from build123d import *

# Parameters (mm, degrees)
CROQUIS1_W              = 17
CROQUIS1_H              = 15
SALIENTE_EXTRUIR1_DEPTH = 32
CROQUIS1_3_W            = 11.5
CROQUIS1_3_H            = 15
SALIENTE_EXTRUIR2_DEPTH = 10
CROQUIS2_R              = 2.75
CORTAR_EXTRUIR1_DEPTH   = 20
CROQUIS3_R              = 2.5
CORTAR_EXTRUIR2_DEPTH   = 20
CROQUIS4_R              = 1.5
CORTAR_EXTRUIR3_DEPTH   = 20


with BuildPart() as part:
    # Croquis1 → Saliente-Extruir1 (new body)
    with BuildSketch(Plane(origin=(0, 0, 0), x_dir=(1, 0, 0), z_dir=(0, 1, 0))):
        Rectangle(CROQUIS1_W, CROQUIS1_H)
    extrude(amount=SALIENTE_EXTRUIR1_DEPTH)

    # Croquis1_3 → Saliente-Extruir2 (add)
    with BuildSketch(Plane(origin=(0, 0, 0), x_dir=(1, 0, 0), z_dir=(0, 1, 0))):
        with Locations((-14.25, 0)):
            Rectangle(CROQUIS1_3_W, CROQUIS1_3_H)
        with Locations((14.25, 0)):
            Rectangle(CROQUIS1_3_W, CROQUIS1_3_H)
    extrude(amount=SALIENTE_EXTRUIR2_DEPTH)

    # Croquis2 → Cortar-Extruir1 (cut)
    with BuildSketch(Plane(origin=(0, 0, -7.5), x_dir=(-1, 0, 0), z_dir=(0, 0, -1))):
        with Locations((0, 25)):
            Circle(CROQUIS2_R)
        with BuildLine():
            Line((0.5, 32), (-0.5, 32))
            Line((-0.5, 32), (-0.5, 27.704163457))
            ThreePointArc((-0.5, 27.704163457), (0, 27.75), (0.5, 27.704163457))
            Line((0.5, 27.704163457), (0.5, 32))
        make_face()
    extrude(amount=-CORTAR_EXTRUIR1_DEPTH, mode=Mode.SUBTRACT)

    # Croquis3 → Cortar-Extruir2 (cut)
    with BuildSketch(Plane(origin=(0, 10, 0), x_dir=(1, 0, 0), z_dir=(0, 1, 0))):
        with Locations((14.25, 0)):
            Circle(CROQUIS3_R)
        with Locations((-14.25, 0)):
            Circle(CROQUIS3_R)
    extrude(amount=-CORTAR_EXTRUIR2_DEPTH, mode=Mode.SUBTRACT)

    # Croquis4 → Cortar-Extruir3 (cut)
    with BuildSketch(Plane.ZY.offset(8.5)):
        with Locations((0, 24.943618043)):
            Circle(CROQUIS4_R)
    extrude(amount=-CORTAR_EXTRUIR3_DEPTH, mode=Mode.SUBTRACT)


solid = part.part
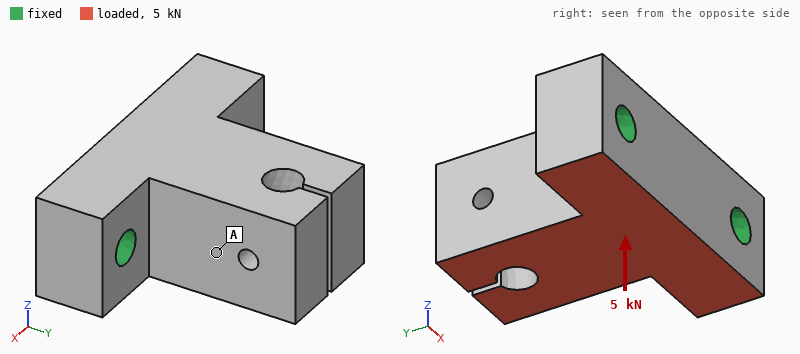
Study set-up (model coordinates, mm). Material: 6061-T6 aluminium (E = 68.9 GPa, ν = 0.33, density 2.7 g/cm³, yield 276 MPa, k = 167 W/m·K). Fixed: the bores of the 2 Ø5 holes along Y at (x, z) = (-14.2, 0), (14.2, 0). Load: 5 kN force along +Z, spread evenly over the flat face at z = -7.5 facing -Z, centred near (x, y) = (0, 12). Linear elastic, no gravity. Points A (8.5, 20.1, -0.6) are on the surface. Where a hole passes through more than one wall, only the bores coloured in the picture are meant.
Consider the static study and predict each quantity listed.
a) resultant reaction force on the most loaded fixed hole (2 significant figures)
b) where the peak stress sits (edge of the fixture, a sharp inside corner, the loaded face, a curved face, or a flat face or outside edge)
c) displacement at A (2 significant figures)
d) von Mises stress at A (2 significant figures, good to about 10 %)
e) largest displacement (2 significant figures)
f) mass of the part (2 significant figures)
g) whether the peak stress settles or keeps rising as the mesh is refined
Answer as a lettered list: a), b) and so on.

a) 2.5 kN
b) edge of the fixture
c) 39 µm
d) 17 MPa
e) 75 µm
f) 29 g
g) keeps rising
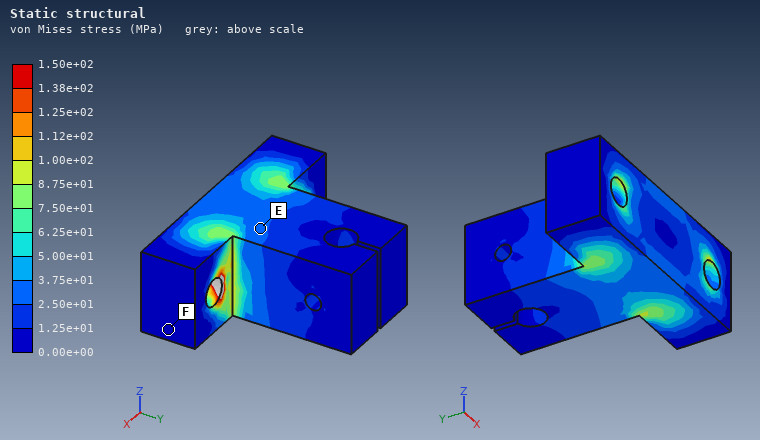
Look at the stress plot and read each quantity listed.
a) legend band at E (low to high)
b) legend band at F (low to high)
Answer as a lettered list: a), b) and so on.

a) 2.50e+01 to 3.75e+01 MPa
b) 0.00e+00 to 1.25e+01 MPa
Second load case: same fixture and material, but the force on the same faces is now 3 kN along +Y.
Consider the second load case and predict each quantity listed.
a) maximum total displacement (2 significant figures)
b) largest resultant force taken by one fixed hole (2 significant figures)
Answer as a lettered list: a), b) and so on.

a) 34 µm
b) 1.5 kN
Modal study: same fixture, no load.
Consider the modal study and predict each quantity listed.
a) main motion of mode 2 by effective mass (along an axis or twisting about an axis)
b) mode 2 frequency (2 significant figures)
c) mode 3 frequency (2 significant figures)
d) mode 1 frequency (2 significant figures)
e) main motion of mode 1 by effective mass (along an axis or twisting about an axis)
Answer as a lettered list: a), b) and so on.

a) along X
b) 15 kHz
c) 24 kHz
d) 9200 Hz
e) along Z
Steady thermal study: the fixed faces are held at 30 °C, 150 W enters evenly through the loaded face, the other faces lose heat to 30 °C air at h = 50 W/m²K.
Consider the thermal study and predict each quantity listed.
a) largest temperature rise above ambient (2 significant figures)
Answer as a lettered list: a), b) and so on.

a) 46 K
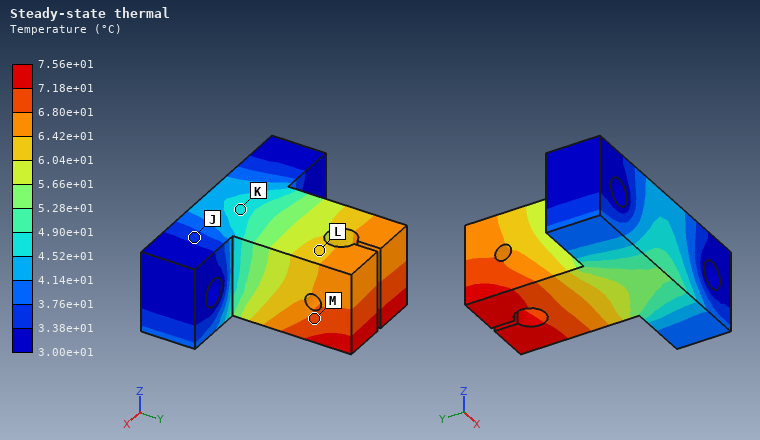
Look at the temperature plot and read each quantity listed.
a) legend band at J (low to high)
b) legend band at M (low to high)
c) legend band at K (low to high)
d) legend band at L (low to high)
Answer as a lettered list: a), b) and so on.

a) 3.38e+01 to 3.76e+01 °C
b) 6.80e+01 to 7.18e+01 °C
c) 4.52e+01 to 4.90e+01 °C
d) 6.04e+01 to 6.42e+01 °C
